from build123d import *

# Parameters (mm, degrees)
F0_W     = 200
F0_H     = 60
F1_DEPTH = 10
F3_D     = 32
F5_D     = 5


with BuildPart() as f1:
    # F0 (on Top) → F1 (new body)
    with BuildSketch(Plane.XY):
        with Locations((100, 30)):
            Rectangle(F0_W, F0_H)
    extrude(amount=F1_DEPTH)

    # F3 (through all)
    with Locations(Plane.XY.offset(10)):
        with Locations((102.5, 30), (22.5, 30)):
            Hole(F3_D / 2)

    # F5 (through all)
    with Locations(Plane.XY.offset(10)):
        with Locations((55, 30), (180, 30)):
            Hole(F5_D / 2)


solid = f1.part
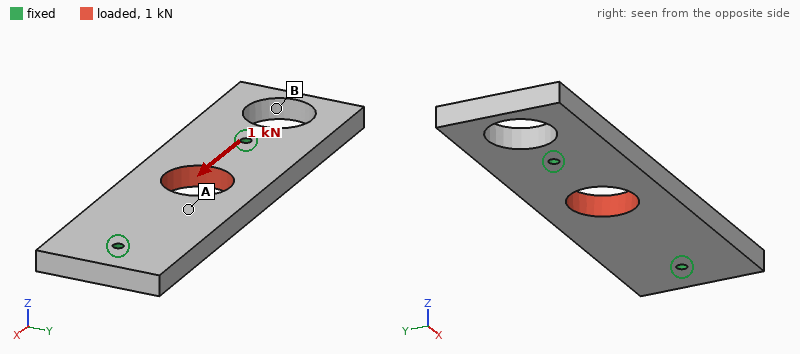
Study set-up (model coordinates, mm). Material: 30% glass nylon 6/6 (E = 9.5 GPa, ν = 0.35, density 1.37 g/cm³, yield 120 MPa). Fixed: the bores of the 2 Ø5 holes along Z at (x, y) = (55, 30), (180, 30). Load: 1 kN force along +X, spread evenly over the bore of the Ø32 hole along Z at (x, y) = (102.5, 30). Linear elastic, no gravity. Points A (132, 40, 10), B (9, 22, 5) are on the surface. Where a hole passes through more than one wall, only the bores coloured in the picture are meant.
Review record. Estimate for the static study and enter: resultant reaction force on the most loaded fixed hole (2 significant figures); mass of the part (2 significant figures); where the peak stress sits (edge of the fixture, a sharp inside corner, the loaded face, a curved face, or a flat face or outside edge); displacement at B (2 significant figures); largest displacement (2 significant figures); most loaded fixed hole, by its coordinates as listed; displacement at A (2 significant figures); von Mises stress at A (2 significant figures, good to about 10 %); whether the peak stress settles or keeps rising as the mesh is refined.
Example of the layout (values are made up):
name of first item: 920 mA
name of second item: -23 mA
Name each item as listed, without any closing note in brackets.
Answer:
resultant reaction force on the most loaded fixed hole: 550 N
mass of the part: 140 g
where the peak stress sits: edge of the fixture
displacement at B: 5.1 µm
largest displacement: 8.9 µm
most loaded fixed hole, by its coordinates as listed: (55, 30)
displacement at A: 6.6 µm
von Mises stress at A: 0.99 MPa
whether the peak stress settles or keeps rising as the mesh is refined: keeps rising
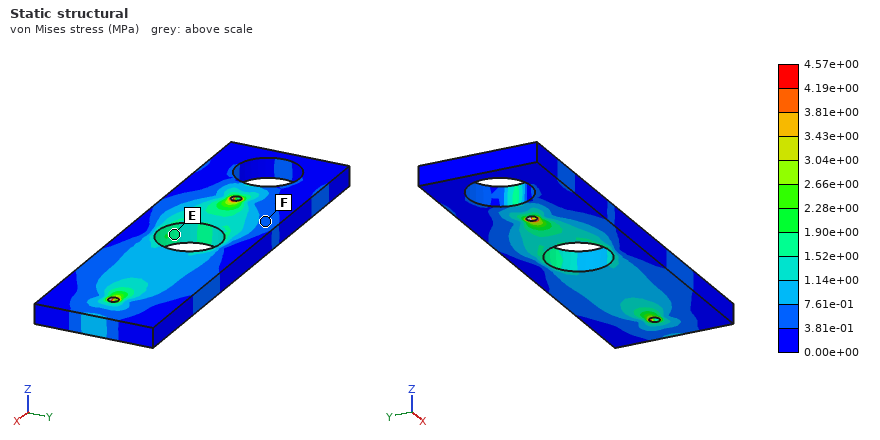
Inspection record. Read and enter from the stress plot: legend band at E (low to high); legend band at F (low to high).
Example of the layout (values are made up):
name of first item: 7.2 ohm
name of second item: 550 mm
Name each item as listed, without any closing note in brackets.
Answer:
legend band at E: 1.52e+00 to 1.90e+00 MPa
legend band at F: 3.81e-01 to 7.61e-01 MPa
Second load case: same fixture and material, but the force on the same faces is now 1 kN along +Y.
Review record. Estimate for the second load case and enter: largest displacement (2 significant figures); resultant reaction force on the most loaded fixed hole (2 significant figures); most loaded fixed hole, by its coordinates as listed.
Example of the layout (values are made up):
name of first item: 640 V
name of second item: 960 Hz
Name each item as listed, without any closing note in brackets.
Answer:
largest displacement: 40 µm
resultant reaction force on the most loaded fixed hole: 620 N
most loaded fixed hole, by its coordinates as listed: (55, 30)
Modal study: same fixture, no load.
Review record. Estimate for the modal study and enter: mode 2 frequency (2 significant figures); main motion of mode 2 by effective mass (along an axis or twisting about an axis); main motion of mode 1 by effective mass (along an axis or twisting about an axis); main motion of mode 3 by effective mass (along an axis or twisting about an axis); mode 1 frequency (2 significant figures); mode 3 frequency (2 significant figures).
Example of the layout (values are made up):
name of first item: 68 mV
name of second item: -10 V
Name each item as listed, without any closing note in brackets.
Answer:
mode 2 frequency: 1500 Hz
main motion of mode 2 by effective mass: along Z
main motion of mode 1 by effective mass: twisting about Y
main motion of mode 3 by effective mass: twisting about X
mode 1 frequency: 1100 Hz
mode 3 frequency: 1600 Hz
